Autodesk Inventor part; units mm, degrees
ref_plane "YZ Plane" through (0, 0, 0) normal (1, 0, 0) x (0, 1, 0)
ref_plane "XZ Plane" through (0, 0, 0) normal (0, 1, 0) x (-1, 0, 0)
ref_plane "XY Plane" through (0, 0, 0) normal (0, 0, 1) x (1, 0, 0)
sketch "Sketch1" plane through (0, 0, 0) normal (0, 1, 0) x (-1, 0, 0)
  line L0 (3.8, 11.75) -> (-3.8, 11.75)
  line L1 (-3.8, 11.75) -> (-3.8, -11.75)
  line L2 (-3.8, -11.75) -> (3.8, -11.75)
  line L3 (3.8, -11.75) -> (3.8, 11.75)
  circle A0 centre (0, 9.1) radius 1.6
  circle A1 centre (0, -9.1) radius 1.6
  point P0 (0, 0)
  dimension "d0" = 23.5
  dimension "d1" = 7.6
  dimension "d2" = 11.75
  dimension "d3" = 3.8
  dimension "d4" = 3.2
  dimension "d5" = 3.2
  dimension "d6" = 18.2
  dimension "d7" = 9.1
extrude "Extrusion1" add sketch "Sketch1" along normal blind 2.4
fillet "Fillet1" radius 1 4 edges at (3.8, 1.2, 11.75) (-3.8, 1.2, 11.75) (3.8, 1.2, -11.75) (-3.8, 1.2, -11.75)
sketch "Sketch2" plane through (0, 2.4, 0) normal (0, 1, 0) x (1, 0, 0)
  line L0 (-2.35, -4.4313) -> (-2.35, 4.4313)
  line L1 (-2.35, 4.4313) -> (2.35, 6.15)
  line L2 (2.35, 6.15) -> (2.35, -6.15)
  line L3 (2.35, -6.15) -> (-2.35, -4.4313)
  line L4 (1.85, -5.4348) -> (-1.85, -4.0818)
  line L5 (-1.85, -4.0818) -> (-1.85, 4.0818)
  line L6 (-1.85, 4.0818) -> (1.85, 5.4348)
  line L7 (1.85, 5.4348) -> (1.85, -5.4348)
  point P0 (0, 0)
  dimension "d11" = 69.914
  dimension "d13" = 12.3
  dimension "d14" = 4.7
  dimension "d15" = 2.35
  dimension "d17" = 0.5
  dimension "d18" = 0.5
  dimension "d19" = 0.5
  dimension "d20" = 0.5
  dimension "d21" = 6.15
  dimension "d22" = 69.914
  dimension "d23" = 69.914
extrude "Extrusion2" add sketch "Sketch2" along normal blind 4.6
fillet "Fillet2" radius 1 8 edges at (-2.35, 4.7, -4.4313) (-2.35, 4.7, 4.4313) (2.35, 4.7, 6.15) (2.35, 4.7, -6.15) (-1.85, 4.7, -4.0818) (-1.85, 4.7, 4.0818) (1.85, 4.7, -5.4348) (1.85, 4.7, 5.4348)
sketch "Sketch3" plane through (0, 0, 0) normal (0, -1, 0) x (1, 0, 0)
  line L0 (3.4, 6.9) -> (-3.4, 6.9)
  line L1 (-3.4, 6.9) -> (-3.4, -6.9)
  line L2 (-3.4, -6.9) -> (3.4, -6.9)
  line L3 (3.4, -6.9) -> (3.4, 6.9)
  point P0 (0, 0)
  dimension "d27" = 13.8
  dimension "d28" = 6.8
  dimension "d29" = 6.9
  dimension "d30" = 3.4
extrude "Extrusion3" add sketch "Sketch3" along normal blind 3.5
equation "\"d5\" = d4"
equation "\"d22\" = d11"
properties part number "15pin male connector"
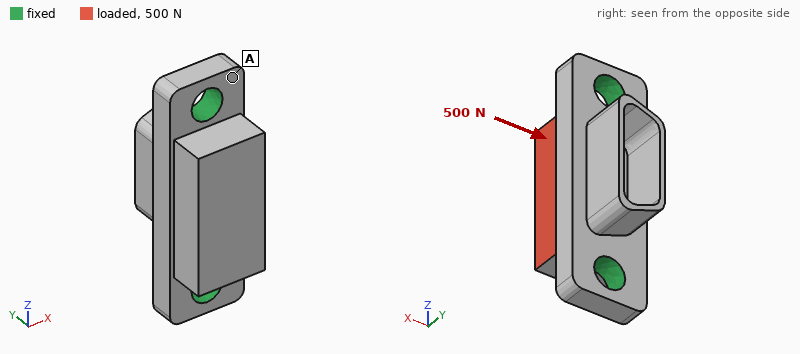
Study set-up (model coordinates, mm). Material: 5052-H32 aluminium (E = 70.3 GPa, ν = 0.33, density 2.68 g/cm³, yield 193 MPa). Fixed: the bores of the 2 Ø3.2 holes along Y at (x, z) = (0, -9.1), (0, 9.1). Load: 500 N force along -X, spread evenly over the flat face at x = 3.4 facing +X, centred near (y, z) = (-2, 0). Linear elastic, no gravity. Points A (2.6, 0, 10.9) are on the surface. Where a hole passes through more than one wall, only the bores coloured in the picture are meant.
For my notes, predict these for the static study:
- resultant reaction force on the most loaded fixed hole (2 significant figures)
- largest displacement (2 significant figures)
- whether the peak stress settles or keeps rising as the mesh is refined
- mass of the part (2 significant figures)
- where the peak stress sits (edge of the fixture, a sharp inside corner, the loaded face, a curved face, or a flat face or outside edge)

250 N
12 µm
keeps rising
2.1 g
edge of the fixture
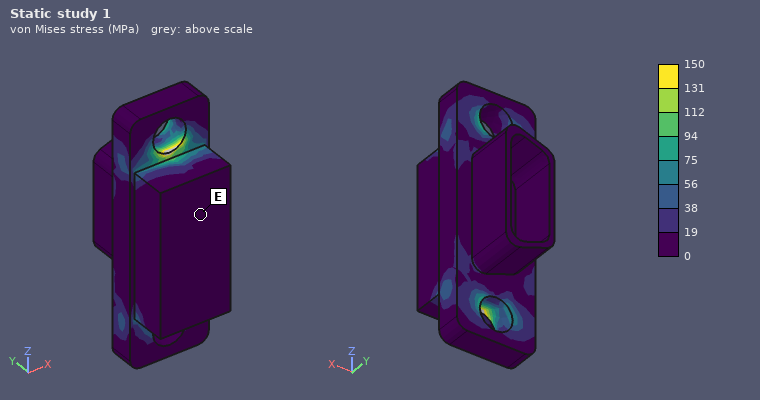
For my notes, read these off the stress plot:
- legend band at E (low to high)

0 to 19 MPa
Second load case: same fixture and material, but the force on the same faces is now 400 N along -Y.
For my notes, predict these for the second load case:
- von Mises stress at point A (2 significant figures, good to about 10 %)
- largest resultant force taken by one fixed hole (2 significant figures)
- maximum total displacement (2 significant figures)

11 MPa
220 N
11 µm
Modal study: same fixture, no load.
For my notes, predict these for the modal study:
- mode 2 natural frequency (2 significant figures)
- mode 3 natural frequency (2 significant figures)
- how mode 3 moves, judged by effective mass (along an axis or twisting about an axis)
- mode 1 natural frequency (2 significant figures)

37 kHz
42 kHz
along X
33 kHz
